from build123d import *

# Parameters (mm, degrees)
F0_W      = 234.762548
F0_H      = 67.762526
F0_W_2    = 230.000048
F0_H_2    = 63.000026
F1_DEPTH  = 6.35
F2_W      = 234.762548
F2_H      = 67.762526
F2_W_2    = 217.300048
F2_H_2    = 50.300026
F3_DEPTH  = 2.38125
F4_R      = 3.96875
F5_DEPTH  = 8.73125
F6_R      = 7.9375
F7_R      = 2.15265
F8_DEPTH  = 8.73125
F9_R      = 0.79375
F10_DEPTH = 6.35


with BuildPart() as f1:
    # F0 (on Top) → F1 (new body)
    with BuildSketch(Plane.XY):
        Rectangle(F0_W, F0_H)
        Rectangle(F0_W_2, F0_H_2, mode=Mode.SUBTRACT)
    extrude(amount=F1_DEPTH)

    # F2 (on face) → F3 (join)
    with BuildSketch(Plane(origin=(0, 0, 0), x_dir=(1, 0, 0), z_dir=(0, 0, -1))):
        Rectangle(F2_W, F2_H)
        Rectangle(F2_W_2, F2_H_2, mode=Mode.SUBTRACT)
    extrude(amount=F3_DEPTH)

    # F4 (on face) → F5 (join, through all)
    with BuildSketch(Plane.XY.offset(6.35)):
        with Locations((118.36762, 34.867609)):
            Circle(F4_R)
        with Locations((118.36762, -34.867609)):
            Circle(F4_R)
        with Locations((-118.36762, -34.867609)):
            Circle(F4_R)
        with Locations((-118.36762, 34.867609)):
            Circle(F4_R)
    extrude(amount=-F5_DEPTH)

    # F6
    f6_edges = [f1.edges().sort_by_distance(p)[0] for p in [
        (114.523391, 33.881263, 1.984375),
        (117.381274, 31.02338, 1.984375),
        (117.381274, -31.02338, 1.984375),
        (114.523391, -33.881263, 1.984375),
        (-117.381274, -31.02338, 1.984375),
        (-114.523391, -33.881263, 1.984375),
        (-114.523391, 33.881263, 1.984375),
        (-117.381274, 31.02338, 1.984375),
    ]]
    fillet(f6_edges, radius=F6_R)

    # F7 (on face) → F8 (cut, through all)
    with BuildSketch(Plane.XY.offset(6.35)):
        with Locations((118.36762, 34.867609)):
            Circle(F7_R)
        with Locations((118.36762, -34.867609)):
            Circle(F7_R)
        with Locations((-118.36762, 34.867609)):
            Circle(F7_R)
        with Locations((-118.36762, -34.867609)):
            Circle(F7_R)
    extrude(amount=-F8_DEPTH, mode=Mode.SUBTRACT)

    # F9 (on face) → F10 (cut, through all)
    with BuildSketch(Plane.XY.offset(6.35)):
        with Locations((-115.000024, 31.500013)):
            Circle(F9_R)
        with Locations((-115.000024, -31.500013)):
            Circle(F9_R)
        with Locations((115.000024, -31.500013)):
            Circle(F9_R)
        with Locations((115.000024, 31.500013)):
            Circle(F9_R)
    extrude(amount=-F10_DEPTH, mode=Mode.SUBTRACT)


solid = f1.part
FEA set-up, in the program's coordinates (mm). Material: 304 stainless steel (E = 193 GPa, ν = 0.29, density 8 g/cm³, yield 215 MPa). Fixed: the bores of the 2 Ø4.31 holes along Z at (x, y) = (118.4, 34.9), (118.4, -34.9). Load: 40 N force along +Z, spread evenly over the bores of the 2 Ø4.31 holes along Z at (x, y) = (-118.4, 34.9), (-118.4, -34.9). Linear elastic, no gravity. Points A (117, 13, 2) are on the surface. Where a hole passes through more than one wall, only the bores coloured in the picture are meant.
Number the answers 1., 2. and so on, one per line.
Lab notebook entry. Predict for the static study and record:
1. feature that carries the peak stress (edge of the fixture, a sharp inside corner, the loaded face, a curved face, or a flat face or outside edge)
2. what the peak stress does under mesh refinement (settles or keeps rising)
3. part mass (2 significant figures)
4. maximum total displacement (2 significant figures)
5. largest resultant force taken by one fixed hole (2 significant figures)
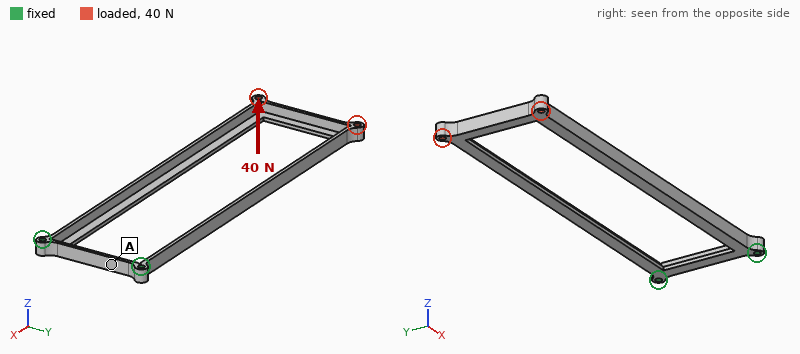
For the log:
1. edge of the fixture
2. keeps rising
3. 180 g
4. 2.0 mm
5. 140 N
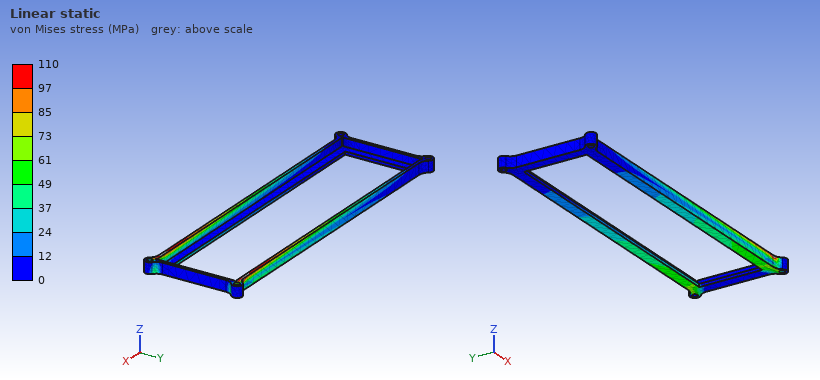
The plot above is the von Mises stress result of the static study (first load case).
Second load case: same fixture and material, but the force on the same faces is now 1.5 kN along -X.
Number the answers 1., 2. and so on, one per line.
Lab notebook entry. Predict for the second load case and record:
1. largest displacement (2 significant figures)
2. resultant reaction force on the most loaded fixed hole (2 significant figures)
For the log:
1. 0.62 mm
2. 760 N
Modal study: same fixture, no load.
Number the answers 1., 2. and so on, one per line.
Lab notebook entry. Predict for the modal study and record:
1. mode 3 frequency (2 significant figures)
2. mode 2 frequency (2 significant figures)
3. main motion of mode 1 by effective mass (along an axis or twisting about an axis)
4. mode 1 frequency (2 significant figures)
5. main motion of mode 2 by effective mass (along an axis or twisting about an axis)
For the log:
1. 220 Hz
2. 140 Hz
3. along Z
4. 98 Hz
5. along Y
